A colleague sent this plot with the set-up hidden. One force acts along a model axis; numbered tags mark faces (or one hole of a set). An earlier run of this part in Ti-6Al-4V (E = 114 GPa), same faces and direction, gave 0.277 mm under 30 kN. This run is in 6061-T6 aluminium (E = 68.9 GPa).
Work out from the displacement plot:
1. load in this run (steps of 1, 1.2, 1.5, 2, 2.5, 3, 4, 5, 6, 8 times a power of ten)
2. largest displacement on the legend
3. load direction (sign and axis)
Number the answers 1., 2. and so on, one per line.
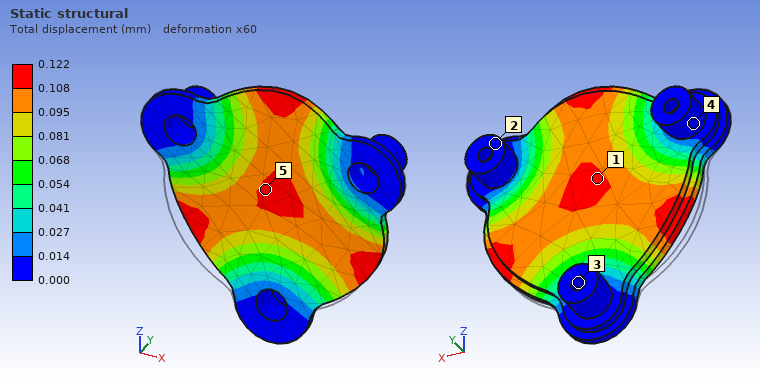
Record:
1. 8 kN
2. 0.122 mm
3. +Y
